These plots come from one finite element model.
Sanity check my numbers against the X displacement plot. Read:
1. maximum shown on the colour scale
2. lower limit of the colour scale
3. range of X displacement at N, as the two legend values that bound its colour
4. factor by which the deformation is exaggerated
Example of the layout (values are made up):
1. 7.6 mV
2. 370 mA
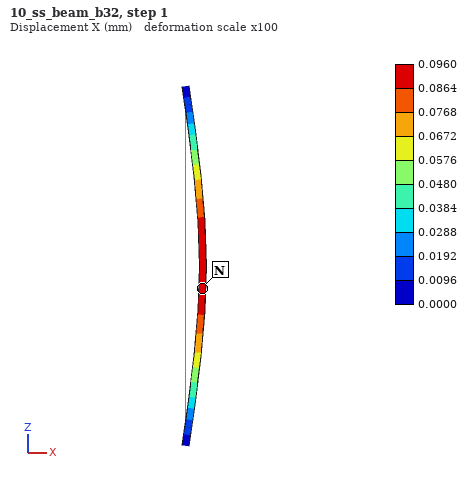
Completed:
1. 0.0960 mm
2. 0.0000 mm
3. 0.0864 to 0.0960 mm
4. 100
